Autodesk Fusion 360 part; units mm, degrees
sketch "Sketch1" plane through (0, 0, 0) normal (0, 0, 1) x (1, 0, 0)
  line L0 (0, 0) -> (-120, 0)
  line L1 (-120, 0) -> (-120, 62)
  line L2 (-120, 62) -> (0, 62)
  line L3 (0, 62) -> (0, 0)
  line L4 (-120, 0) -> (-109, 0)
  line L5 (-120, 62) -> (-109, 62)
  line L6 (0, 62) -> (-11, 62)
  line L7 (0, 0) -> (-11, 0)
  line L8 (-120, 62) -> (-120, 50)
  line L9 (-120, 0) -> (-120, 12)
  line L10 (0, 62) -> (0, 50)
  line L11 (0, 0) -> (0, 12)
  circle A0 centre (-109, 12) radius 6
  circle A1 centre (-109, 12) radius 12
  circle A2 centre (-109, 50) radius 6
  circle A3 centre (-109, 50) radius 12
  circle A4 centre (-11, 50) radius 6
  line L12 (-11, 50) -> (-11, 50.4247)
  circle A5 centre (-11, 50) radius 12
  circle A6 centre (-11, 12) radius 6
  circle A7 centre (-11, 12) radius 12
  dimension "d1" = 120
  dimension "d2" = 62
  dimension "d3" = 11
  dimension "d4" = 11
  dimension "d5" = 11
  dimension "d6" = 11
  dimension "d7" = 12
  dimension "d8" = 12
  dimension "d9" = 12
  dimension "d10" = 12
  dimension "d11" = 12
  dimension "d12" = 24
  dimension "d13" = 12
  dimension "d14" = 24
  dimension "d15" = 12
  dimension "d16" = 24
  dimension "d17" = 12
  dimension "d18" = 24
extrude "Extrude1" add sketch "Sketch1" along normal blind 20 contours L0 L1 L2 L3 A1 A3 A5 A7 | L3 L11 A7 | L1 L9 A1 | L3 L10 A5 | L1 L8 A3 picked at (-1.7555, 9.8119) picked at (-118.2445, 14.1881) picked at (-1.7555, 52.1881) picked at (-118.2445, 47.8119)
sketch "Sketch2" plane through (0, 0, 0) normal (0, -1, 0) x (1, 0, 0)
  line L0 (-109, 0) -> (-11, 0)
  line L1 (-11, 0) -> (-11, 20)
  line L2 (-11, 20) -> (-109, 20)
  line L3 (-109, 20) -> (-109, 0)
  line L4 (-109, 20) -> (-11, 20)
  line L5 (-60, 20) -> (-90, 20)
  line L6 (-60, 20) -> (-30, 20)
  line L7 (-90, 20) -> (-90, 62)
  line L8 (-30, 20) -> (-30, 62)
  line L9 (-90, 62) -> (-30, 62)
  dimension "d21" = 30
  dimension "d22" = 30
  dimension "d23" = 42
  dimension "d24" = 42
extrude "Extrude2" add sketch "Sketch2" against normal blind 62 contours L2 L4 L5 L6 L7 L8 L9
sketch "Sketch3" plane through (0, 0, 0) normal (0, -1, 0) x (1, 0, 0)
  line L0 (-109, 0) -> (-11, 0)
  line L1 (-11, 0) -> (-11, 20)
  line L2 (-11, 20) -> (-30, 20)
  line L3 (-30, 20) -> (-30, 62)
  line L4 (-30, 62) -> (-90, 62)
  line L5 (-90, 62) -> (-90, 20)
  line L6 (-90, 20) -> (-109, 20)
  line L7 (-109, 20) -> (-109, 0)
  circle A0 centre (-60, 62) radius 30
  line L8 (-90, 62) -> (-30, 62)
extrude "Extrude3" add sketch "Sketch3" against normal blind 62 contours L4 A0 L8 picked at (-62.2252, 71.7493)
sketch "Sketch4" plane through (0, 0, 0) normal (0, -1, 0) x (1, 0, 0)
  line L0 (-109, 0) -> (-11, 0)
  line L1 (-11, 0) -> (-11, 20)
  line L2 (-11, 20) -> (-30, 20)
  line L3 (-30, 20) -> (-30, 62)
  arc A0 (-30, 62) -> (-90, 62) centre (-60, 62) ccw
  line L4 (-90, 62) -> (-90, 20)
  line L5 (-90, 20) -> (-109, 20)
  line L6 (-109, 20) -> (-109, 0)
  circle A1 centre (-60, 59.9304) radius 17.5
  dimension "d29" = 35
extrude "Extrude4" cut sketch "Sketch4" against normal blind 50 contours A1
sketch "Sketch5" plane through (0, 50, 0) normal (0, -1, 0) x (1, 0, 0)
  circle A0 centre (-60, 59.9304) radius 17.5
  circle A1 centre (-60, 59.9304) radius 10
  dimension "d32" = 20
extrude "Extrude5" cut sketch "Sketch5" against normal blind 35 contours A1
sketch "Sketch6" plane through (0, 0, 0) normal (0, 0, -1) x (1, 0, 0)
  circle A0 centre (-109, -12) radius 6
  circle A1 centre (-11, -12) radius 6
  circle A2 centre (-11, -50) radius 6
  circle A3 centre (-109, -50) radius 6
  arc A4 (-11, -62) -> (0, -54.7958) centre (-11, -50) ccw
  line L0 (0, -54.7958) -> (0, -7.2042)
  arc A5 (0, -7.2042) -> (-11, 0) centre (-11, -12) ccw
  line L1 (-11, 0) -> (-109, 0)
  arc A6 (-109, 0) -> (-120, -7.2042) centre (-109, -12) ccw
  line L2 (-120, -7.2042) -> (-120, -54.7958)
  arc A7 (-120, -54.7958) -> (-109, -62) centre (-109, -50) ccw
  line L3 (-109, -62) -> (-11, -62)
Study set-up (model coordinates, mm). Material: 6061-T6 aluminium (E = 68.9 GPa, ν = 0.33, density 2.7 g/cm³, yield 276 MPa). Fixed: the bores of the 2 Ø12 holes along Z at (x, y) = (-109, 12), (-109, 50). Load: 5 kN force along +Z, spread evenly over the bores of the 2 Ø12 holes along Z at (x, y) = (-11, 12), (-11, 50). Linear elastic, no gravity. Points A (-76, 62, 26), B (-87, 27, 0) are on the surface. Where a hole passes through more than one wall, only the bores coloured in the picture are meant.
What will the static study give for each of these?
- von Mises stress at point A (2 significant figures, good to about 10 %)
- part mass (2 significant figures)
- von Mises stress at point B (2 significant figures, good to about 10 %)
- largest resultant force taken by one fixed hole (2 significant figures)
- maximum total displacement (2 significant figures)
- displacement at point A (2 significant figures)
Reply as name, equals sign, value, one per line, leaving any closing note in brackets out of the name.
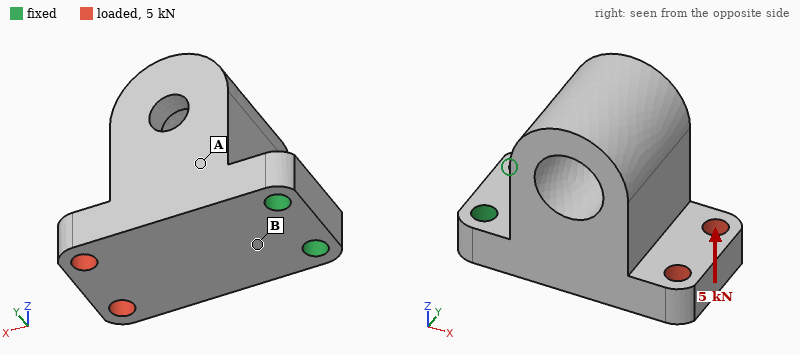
von Mises stress at point A = 21 MPa
part mass = 890 g
von Mises stress at point B = 66 MPa
largest resultant force taken by one fixed hole = 2.5 kN
maximum total displacement = 0.42 mm
displacement at point A = 0.095 mm
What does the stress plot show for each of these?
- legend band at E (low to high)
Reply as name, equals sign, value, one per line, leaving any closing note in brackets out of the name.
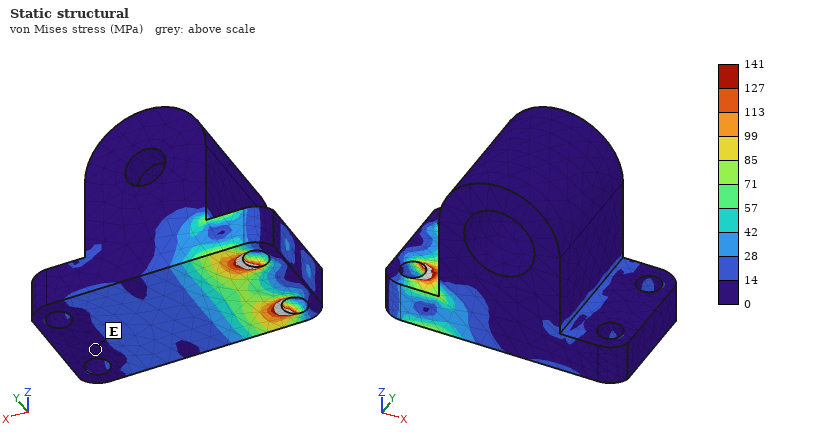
legend band at E = 0 to 14 MPa
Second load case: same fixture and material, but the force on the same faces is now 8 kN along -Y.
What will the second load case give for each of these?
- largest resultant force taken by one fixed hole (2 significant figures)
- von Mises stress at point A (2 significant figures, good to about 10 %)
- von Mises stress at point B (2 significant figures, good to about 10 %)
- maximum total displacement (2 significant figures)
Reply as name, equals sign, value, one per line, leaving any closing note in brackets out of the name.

largest resultant force taken by one fixed hole = 18 kN
von Mises stress at point A = 15 MPa
von Mises stress at point B = 25 MPa
maximum total displacement = 0.12 mm
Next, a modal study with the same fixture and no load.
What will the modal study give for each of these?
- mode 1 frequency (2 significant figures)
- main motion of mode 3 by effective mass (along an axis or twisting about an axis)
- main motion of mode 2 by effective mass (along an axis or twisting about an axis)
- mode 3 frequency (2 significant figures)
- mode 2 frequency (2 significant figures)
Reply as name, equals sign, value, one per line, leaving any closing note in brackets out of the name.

mode 1 frequency = 980 Hz
main motion of mode 3 by effective mass = along Y
main motion of mode 2 by effective mass = along Y
mode 3 frequency = 3300 Hz
mode 2 frequency = 2200 Hz
